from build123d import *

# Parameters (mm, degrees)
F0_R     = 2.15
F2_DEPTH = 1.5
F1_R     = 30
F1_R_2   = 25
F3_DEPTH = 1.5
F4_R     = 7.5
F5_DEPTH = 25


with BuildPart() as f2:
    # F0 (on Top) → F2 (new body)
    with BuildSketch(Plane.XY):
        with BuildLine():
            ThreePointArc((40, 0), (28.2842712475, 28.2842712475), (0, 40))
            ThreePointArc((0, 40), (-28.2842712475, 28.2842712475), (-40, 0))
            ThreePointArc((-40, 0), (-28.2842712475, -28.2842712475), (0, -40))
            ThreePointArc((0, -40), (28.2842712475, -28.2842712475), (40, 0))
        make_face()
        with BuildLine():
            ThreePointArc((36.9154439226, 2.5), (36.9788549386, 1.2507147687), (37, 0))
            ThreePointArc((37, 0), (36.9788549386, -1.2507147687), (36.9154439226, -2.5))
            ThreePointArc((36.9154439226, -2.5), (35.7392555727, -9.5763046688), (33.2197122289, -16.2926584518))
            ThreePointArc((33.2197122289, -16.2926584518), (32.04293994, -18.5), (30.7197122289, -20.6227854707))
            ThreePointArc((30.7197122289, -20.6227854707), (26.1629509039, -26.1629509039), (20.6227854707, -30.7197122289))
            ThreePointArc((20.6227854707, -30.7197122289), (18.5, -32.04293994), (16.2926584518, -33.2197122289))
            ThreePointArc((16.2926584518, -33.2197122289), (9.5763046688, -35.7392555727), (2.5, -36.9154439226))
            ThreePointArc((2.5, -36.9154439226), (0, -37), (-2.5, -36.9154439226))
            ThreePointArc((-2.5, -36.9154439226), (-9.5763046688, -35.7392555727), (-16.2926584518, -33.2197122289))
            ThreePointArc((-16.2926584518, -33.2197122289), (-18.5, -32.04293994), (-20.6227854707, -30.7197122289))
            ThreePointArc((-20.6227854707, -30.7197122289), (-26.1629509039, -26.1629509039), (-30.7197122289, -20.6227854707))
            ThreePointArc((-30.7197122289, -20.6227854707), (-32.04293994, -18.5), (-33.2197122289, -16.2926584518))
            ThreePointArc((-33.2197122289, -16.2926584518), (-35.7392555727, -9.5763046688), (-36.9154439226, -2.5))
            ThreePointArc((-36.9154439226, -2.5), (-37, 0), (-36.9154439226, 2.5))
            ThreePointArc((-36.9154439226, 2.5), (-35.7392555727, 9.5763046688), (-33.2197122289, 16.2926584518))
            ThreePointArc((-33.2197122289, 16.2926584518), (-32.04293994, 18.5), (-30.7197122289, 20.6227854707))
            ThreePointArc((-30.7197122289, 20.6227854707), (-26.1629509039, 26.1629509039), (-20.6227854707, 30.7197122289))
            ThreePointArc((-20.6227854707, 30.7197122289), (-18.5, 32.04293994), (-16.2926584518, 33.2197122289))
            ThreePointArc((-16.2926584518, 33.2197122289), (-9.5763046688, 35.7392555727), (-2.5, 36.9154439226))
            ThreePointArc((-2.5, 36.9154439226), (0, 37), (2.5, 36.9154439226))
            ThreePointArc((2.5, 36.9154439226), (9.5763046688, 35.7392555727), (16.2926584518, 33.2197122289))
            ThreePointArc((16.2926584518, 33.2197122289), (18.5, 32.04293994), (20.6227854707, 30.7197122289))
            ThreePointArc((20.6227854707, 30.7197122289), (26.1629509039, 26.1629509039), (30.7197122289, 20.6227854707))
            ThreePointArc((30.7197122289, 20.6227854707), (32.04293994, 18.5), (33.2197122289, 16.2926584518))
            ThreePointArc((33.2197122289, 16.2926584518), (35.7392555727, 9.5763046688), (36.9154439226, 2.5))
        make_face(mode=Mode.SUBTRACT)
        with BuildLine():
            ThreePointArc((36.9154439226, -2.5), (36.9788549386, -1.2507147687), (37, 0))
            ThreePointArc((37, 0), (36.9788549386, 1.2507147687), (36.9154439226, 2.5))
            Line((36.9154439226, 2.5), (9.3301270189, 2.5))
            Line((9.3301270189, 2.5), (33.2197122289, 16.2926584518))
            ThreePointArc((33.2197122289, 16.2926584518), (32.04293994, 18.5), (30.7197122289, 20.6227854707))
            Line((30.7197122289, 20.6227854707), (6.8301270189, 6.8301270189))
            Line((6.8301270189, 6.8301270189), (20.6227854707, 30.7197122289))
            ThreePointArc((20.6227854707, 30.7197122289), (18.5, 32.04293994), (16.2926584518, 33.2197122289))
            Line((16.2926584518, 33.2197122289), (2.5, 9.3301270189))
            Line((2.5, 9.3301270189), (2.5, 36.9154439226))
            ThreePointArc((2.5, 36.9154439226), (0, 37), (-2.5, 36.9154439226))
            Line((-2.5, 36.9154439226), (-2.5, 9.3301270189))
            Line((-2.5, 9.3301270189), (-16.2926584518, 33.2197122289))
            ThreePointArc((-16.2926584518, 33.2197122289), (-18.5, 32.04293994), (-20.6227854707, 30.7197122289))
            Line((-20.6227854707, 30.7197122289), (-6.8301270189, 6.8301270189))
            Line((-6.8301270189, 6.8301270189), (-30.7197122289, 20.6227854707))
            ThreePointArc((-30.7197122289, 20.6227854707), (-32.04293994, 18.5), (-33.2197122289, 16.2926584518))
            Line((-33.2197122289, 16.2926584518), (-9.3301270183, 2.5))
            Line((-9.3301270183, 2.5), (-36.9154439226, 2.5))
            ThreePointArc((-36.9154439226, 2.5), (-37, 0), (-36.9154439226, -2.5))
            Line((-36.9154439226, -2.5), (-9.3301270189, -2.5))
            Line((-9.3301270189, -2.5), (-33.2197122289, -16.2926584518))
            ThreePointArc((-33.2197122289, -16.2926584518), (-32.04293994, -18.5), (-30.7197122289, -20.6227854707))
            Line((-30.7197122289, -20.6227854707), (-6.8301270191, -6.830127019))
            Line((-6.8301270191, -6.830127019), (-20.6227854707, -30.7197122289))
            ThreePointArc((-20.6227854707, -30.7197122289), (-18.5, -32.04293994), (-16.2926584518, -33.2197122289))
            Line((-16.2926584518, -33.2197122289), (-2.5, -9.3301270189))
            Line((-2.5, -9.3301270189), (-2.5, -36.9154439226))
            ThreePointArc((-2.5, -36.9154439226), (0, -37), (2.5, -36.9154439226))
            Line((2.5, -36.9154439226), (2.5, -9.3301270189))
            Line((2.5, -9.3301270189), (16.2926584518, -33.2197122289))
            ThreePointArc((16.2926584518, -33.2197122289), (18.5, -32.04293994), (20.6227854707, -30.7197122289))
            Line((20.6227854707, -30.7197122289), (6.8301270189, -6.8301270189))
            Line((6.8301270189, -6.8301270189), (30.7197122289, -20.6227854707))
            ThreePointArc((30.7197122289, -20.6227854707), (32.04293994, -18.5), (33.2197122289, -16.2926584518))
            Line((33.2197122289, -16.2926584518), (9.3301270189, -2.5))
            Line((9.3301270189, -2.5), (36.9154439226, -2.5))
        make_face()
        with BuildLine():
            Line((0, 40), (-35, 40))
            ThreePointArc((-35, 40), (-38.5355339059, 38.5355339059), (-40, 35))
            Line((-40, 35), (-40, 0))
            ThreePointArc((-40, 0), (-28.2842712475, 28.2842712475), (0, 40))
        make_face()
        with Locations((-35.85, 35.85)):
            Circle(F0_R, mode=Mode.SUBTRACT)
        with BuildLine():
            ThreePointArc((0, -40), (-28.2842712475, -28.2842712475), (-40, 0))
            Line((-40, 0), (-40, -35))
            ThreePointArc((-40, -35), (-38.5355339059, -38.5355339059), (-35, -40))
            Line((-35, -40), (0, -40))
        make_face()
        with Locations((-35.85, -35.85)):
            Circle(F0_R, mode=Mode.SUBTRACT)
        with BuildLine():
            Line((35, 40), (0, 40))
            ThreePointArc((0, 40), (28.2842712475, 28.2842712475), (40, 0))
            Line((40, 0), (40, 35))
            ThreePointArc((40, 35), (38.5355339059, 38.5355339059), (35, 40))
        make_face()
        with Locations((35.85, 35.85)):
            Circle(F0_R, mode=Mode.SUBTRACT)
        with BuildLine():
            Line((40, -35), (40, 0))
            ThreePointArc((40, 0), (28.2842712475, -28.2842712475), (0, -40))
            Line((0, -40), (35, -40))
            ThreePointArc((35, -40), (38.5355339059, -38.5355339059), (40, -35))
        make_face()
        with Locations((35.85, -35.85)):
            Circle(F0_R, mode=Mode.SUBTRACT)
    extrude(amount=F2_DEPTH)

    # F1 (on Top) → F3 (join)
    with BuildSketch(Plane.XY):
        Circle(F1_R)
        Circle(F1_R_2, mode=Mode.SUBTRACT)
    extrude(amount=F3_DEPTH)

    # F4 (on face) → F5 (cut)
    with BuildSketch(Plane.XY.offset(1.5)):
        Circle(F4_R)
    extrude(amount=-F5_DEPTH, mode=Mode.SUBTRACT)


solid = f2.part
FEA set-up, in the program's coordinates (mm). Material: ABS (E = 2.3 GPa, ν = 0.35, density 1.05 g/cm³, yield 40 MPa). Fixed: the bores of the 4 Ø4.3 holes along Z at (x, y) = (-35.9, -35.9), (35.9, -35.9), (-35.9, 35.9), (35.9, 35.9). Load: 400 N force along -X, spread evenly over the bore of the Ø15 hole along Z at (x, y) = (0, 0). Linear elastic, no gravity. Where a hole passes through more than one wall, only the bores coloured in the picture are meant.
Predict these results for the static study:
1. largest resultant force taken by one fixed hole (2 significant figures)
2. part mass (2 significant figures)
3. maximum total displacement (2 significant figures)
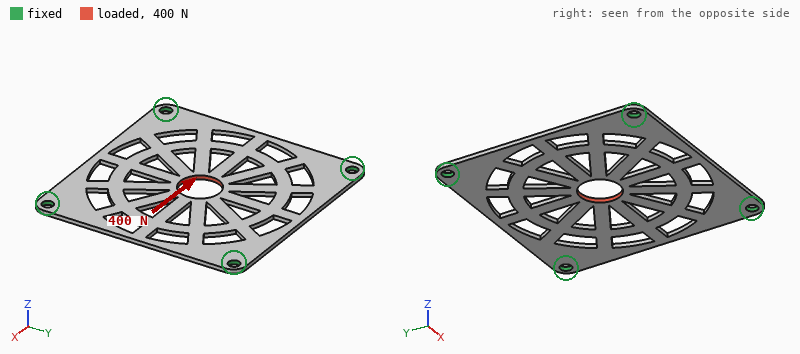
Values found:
110 N
6.8 g
0.27 mm
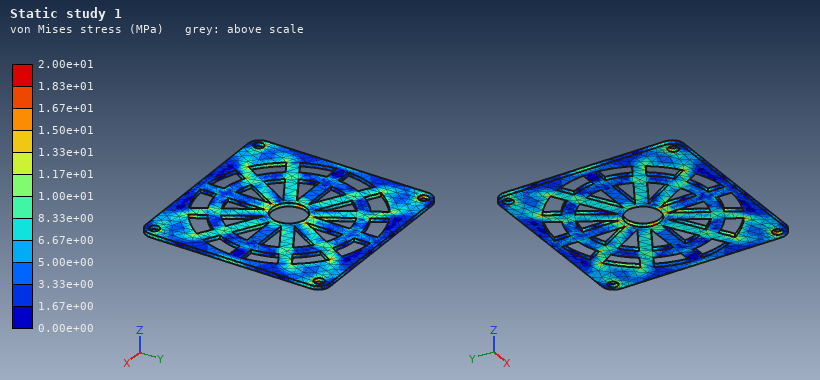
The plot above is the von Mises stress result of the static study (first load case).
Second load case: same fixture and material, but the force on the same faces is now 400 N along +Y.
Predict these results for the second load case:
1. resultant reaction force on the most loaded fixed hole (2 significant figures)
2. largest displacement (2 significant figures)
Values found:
110 N
0.27 mm
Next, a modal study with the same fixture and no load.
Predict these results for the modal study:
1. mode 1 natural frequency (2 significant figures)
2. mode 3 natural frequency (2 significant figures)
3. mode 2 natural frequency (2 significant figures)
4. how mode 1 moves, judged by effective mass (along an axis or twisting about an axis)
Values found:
270 Hz
510 Hz
510 Hz
along Z
